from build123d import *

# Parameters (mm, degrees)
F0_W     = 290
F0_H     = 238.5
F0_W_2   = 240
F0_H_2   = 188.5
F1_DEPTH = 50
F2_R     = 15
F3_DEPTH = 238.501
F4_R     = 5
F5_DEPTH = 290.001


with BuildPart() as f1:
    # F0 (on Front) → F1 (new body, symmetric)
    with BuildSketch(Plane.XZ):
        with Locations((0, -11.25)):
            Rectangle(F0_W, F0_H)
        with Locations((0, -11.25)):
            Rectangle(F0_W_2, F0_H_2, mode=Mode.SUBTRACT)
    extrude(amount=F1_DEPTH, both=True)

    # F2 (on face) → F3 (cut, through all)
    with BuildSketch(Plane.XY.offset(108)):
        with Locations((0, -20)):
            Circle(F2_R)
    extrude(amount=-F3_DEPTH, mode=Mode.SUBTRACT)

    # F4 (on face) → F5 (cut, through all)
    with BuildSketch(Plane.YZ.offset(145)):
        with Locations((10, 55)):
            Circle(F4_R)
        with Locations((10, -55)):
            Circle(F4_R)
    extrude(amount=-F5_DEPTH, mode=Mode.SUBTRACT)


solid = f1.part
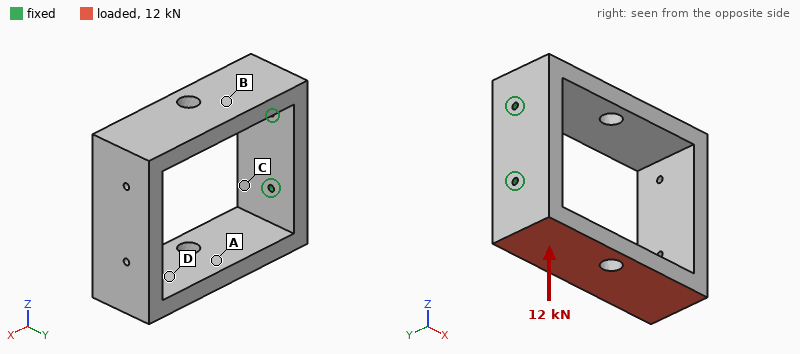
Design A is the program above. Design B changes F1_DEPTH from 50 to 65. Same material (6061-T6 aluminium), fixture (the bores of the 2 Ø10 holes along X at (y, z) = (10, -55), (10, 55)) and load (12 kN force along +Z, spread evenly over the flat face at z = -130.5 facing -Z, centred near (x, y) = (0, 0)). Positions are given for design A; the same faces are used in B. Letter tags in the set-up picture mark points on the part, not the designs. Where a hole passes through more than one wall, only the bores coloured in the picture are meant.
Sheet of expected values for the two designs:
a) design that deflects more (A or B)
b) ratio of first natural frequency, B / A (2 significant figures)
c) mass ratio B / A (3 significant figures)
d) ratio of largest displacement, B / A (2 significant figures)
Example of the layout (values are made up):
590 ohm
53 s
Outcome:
A
0.99
1.31
0.79
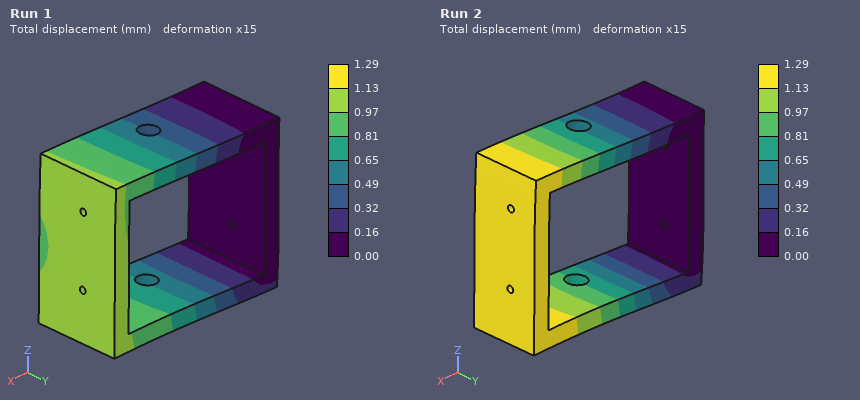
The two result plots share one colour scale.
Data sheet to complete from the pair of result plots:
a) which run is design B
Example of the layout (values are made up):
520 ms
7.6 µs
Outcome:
Run 1
